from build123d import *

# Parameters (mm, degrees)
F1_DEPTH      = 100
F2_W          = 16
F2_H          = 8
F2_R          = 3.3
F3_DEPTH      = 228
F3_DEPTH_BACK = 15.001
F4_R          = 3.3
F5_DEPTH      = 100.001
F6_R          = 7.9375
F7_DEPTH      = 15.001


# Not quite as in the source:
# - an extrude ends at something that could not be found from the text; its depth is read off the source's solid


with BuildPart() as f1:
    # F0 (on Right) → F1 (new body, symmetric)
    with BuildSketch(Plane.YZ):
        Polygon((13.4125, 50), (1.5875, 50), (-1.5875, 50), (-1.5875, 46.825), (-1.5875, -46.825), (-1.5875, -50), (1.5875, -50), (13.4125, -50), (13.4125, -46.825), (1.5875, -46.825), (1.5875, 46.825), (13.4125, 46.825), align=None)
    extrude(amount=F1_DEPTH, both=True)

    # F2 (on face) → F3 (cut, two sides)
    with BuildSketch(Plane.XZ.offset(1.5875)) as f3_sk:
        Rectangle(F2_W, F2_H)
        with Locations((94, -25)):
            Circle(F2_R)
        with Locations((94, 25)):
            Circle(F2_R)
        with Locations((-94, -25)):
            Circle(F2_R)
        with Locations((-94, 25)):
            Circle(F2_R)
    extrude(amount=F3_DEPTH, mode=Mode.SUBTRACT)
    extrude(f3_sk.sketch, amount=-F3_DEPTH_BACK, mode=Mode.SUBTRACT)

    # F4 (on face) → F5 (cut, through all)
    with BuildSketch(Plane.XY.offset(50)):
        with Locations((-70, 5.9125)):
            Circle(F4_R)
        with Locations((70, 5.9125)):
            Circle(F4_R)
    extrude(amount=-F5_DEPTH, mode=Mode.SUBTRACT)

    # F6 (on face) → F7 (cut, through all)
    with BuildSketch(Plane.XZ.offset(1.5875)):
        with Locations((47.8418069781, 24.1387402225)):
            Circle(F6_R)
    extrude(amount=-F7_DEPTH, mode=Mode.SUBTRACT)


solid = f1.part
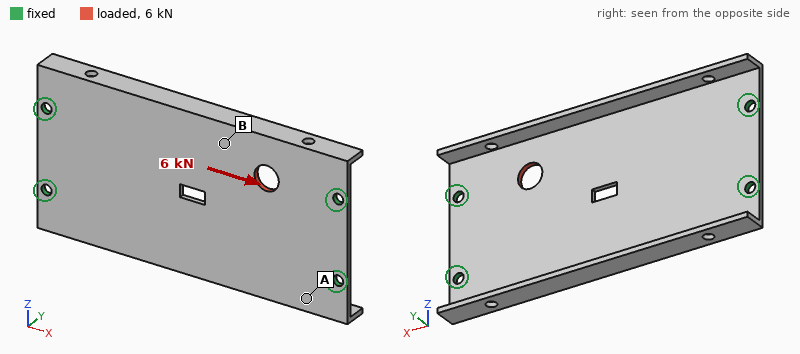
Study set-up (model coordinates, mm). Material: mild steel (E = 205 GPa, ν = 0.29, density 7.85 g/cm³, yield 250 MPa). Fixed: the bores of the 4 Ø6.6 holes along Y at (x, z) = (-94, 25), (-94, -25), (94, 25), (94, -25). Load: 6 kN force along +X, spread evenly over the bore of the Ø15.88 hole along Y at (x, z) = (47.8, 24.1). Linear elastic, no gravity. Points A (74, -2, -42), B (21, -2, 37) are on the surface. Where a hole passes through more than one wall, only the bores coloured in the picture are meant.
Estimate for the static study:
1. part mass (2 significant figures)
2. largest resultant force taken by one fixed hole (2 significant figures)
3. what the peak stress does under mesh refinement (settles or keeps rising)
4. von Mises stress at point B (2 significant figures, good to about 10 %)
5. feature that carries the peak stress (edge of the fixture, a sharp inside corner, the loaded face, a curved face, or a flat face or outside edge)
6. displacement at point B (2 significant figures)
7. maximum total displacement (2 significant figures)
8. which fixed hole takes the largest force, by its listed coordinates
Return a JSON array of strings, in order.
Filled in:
["600 g", "3.0 kN", "keeps rising", "16 MPa", "edge of the fixture", "9.9 µm", "13 µm", "(94, 25)"]
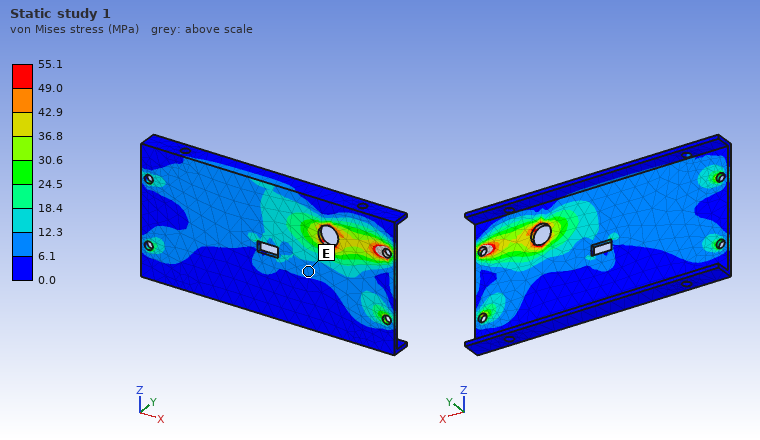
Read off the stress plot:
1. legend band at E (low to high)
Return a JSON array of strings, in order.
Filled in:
["6.1 to 12.3 MPa"]
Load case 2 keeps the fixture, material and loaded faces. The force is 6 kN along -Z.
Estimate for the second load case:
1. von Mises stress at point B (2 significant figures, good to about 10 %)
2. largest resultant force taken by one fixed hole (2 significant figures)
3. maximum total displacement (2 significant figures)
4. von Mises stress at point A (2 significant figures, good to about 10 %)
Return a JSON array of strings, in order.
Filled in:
["16 MPa", "2.6 kN", "35 µm", "8.7 MPa"]
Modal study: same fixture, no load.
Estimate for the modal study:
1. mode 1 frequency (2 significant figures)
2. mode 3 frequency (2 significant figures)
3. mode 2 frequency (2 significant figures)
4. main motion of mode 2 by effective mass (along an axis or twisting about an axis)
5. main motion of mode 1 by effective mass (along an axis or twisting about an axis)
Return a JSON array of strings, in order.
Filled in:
["790 Hz", "1500 Hz", "950 Hz", "twisting about X", "along Y"]
